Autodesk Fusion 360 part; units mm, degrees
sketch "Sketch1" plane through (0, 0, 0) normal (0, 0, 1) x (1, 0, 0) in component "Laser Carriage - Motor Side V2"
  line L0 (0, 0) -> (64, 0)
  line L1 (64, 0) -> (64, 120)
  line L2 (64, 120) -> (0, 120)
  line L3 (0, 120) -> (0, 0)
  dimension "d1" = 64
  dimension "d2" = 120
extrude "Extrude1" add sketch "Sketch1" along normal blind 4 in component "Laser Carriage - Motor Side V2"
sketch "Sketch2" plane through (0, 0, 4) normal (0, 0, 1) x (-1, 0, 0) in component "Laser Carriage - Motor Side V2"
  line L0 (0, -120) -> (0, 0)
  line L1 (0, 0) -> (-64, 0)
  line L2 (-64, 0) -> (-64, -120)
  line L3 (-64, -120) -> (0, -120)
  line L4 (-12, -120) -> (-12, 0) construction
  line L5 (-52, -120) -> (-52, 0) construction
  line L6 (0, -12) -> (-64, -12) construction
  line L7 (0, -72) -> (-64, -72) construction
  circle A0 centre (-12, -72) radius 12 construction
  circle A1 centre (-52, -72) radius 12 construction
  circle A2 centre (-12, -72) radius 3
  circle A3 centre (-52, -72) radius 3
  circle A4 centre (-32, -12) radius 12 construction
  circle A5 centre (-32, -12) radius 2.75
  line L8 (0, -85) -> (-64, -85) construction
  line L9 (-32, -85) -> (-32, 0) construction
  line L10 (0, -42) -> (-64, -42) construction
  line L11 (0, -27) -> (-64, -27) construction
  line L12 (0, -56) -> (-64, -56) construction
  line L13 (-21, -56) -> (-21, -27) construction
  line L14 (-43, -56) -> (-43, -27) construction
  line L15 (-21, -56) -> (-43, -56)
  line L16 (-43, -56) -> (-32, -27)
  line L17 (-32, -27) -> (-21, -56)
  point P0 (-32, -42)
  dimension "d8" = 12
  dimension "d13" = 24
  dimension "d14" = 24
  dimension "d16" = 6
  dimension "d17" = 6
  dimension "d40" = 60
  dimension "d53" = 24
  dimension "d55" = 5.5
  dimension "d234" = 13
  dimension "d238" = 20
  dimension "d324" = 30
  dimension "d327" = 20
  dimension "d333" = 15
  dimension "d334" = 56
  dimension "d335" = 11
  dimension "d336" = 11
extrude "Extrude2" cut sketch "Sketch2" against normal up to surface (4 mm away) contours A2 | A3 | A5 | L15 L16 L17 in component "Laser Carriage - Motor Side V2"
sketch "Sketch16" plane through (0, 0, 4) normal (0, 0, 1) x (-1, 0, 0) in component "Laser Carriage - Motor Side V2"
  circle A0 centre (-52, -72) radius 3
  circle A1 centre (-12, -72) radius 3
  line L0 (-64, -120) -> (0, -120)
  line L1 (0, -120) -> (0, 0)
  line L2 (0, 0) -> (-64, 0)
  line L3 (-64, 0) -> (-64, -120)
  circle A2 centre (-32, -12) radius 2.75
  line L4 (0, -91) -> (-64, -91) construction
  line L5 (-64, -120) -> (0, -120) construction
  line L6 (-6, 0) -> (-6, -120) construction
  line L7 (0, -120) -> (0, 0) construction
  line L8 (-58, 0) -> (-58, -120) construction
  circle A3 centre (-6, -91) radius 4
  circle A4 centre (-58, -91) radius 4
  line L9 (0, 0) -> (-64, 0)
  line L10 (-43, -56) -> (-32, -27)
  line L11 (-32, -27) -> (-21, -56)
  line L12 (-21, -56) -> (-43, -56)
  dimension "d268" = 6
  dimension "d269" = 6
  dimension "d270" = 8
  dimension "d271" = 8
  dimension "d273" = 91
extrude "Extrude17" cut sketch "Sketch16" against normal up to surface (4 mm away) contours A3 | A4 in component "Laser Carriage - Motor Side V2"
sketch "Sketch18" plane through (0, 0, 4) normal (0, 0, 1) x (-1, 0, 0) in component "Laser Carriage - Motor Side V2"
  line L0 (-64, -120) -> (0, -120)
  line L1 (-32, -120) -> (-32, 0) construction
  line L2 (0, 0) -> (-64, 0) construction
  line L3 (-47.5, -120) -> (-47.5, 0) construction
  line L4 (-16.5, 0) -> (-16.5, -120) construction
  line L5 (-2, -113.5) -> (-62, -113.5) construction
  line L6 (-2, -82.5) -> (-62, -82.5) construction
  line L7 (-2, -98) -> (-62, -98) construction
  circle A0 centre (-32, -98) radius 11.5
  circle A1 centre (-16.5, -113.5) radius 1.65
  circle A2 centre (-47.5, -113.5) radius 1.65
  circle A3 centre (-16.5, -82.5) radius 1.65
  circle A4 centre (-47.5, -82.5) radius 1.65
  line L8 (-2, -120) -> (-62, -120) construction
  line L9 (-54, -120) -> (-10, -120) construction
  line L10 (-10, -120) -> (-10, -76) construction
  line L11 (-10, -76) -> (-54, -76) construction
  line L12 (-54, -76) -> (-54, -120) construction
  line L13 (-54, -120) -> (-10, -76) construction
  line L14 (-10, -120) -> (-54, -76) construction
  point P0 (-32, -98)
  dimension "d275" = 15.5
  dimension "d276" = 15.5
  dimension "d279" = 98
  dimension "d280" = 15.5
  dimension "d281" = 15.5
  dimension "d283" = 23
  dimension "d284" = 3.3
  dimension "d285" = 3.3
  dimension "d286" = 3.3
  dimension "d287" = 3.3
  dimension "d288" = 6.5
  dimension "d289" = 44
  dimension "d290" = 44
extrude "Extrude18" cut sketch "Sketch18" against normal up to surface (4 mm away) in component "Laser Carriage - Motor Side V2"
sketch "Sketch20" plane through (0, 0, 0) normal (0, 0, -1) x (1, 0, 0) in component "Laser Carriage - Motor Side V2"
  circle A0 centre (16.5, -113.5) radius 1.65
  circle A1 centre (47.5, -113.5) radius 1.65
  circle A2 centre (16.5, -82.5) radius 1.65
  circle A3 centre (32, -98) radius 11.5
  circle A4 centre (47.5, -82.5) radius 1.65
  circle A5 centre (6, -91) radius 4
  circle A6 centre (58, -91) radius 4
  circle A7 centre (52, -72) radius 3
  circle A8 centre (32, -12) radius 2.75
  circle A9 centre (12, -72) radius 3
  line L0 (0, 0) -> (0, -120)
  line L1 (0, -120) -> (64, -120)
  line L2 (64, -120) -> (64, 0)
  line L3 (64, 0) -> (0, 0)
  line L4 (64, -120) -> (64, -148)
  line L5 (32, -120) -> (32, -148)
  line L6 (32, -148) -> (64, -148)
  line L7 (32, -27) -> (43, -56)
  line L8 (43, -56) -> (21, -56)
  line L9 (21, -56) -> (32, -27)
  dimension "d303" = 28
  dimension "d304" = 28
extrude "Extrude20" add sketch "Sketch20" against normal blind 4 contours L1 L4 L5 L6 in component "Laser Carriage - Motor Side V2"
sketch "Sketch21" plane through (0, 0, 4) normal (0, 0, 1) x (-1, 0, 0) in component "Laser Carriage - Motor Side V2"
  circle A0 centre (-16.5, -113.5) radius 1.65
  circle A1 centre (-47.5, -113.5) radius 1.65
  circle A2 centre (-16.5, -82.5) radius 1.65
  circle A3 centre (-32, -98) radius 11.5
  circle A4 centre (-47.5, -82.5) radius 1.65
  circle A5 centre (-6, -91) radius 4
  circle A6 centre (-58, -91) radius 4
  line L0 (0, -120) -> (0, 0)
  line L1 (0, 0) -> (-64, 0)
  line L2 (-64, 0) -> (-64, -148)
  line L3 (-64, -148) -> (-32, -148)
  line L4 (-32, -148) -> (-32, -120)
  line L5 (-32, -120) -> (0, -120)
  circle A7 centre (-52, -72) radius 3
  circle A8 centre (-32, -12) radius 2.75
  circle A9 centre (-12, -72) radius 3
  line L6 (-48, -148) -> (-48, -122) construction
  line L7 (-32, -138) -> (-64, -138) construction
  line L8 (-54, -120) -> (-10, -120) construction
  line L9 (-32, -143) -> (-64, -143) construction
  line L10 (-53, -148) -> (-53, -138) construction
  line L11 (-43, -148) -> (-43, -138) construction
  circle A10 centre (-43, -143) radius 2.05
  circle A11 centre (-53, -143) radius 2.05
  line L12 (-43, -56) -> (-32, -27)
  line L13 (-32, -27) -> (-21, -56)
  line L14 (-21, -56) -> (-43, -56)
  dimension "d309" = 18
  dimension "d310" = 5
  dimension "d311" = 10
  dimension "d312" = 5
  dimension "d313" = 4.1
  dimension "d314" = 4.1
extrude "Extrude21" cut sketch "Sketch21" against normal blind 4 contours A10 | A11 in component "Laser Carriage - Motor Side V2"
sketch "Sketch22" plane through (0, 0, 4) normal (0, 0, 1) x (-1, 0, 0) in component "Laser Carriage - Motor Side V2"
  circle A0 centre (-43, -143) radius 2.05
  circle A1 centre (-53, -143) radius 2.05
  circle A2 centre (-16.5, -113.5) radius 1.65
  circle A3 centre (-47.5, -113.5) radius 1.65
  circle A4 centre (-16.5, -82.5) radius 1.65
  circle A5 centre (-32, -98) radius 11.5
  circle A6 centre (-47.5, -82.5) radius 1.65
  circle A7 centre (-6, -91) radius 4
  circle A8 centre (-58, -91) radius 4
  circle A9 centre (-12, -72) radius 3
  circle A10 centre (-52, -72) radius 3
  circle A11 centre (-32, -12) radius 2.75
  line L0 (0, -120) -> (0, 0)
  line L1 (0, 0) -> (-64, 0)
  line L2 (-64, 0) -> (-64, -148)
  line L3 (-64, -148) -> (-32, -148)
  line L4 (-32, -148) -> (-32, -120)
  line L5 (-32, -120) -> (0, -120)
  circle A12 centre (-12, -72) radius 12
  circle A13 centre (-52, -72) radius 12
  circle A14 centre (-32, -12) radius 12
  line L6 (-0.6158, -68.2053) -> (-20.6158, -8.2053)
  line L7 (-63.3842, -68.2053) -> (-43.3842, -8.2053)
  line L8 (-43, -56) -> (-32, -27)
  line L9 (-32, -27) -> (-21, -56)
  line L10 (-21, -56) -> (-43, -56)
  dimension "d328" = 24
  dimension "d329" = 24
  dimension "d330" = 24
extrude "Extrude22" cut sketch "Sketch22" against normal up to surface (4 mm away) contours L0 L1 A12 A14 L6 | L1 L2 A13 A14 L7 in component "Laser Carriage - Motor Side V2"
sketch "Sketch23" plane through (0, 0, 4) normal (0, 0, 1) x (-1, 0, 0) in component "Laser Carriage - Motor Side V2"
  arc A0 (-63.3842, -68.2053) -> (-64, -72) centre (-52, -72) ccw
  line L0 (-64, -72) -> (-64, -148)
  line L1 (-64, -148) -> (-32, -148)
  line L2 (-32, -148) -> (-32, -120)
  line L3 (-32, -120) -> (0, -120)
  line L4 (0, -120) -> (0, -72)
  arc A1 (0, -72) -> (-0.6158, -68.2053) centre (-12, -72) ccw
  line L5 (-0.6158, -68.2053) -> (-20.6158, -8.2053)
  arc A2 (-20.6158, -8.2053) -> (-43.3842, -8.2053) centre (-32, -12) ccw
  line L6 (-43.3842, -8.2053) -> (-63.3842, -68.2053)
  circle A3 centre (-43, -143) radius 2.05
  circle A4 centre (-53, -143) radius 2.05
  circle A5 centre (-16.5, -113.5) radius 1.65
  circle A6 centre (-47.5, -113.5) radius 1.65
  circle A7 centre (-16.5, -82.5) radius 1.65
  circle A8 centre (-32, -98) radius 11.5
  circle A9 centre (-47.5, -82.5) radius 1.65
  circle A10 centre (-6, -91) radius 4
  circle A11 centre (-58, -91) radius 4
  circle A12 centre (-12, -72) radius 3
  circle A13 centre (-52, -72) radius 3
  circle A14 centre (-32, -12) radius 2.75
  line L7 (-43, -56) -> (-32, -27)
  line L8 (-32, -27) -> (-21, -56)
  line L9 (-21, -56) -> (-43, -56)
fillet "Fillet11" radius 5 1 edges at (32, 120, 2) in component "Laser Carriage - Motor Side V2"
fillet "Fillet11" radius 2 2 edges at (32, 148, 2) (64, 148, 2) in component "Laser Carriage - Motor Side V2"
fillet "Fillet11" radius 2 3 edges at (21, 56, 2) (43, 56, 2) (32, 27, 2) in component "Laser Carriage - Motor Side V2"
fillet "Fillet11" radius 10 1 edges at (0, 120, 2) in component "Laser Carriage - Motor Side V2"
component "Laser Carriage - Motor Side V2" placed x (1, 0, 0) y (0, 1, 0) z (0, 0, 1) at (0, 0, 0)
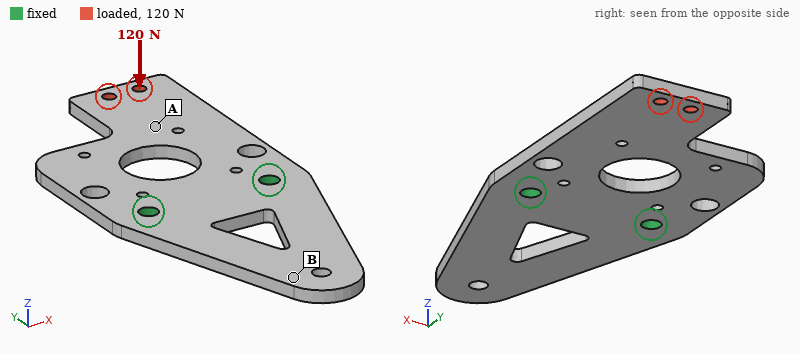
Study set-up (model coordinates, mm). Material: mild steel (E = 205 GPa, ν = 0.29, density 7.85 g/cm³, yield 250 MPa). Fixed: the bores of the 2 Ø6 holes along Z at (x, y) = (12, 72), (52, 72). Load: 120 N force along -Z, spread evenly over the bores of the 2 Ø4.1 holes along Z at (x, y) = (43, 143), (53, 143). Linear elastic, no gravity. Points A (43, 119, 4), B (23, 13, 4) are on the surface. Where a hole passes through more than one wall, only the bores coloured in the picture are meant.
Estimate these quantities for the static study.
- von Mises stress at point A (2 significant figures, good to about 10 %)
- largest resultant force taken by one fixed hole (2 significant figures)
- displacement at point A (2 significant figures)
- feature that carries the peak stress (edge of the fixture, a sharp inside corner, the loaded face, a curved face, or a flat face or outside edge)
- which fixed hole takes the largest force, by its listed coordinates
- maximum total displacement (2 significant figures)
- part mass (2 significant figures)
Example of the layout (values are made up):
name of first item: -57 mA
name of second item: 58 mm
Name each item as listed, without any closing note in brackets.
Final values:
von Mises stress at point A: 32 MPa
largest resultant force taken by one fixed hole: 96 N
displacement at point A: 0.17 mm
feature that carries the peak stress: a curved face
which fixed hole takes the largest force, by its listed coordinates: (52, 72)
maximum total displacement: 0.40 mm
part mass: 190 g
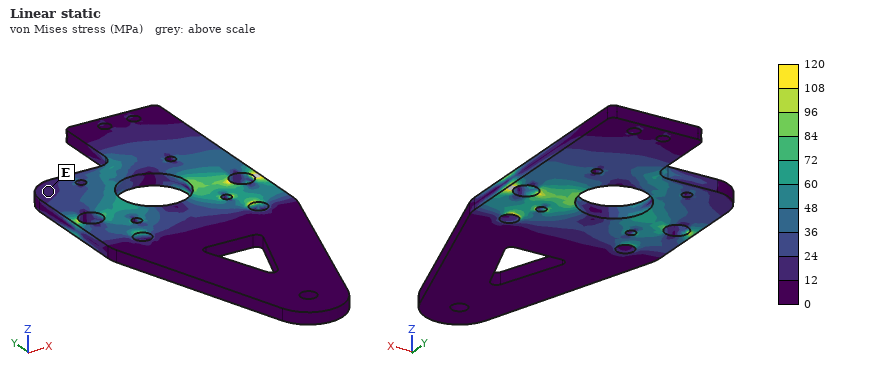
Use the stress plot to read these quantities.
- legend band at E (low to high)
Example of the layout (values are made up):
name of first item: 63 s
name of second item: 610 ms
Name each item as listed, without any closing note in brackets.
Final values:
legend band at E: 12 to 24 MPa
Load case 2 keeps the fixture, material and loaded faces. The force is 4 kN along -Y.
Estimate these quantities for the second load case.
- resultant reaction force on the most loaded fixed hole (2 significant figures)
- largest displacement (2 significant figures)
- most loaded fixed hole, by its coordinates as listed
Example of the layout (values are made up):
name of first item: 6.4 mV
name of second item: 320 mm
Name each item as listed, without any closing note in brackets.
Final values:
resultant reaction force on the most loaded fixed hole: 3.5 kN
largest displacement: 20 µm
most loaded fixed hole, by its coordinates as listed: (52, 72)
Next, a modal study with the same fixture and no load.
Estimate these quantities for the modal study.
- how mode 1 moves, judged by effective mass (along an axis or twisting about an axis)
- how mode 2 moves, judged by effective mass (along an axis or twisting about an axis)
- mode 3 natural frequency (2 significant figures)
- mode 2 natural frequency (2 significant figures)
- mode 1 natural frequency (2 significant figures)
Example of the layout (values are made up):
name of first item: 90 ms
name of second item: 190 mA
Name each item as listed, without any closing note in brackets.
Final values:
how mode 1 moves, judged by effective mass: along Z
how mode 2 moves, judged by effective mass: along Z
mode 3 natural frequency: 2100 Hz
mode 2 natural frequency: 860 Hz
mode 1 natural frequency: 630 Hz
